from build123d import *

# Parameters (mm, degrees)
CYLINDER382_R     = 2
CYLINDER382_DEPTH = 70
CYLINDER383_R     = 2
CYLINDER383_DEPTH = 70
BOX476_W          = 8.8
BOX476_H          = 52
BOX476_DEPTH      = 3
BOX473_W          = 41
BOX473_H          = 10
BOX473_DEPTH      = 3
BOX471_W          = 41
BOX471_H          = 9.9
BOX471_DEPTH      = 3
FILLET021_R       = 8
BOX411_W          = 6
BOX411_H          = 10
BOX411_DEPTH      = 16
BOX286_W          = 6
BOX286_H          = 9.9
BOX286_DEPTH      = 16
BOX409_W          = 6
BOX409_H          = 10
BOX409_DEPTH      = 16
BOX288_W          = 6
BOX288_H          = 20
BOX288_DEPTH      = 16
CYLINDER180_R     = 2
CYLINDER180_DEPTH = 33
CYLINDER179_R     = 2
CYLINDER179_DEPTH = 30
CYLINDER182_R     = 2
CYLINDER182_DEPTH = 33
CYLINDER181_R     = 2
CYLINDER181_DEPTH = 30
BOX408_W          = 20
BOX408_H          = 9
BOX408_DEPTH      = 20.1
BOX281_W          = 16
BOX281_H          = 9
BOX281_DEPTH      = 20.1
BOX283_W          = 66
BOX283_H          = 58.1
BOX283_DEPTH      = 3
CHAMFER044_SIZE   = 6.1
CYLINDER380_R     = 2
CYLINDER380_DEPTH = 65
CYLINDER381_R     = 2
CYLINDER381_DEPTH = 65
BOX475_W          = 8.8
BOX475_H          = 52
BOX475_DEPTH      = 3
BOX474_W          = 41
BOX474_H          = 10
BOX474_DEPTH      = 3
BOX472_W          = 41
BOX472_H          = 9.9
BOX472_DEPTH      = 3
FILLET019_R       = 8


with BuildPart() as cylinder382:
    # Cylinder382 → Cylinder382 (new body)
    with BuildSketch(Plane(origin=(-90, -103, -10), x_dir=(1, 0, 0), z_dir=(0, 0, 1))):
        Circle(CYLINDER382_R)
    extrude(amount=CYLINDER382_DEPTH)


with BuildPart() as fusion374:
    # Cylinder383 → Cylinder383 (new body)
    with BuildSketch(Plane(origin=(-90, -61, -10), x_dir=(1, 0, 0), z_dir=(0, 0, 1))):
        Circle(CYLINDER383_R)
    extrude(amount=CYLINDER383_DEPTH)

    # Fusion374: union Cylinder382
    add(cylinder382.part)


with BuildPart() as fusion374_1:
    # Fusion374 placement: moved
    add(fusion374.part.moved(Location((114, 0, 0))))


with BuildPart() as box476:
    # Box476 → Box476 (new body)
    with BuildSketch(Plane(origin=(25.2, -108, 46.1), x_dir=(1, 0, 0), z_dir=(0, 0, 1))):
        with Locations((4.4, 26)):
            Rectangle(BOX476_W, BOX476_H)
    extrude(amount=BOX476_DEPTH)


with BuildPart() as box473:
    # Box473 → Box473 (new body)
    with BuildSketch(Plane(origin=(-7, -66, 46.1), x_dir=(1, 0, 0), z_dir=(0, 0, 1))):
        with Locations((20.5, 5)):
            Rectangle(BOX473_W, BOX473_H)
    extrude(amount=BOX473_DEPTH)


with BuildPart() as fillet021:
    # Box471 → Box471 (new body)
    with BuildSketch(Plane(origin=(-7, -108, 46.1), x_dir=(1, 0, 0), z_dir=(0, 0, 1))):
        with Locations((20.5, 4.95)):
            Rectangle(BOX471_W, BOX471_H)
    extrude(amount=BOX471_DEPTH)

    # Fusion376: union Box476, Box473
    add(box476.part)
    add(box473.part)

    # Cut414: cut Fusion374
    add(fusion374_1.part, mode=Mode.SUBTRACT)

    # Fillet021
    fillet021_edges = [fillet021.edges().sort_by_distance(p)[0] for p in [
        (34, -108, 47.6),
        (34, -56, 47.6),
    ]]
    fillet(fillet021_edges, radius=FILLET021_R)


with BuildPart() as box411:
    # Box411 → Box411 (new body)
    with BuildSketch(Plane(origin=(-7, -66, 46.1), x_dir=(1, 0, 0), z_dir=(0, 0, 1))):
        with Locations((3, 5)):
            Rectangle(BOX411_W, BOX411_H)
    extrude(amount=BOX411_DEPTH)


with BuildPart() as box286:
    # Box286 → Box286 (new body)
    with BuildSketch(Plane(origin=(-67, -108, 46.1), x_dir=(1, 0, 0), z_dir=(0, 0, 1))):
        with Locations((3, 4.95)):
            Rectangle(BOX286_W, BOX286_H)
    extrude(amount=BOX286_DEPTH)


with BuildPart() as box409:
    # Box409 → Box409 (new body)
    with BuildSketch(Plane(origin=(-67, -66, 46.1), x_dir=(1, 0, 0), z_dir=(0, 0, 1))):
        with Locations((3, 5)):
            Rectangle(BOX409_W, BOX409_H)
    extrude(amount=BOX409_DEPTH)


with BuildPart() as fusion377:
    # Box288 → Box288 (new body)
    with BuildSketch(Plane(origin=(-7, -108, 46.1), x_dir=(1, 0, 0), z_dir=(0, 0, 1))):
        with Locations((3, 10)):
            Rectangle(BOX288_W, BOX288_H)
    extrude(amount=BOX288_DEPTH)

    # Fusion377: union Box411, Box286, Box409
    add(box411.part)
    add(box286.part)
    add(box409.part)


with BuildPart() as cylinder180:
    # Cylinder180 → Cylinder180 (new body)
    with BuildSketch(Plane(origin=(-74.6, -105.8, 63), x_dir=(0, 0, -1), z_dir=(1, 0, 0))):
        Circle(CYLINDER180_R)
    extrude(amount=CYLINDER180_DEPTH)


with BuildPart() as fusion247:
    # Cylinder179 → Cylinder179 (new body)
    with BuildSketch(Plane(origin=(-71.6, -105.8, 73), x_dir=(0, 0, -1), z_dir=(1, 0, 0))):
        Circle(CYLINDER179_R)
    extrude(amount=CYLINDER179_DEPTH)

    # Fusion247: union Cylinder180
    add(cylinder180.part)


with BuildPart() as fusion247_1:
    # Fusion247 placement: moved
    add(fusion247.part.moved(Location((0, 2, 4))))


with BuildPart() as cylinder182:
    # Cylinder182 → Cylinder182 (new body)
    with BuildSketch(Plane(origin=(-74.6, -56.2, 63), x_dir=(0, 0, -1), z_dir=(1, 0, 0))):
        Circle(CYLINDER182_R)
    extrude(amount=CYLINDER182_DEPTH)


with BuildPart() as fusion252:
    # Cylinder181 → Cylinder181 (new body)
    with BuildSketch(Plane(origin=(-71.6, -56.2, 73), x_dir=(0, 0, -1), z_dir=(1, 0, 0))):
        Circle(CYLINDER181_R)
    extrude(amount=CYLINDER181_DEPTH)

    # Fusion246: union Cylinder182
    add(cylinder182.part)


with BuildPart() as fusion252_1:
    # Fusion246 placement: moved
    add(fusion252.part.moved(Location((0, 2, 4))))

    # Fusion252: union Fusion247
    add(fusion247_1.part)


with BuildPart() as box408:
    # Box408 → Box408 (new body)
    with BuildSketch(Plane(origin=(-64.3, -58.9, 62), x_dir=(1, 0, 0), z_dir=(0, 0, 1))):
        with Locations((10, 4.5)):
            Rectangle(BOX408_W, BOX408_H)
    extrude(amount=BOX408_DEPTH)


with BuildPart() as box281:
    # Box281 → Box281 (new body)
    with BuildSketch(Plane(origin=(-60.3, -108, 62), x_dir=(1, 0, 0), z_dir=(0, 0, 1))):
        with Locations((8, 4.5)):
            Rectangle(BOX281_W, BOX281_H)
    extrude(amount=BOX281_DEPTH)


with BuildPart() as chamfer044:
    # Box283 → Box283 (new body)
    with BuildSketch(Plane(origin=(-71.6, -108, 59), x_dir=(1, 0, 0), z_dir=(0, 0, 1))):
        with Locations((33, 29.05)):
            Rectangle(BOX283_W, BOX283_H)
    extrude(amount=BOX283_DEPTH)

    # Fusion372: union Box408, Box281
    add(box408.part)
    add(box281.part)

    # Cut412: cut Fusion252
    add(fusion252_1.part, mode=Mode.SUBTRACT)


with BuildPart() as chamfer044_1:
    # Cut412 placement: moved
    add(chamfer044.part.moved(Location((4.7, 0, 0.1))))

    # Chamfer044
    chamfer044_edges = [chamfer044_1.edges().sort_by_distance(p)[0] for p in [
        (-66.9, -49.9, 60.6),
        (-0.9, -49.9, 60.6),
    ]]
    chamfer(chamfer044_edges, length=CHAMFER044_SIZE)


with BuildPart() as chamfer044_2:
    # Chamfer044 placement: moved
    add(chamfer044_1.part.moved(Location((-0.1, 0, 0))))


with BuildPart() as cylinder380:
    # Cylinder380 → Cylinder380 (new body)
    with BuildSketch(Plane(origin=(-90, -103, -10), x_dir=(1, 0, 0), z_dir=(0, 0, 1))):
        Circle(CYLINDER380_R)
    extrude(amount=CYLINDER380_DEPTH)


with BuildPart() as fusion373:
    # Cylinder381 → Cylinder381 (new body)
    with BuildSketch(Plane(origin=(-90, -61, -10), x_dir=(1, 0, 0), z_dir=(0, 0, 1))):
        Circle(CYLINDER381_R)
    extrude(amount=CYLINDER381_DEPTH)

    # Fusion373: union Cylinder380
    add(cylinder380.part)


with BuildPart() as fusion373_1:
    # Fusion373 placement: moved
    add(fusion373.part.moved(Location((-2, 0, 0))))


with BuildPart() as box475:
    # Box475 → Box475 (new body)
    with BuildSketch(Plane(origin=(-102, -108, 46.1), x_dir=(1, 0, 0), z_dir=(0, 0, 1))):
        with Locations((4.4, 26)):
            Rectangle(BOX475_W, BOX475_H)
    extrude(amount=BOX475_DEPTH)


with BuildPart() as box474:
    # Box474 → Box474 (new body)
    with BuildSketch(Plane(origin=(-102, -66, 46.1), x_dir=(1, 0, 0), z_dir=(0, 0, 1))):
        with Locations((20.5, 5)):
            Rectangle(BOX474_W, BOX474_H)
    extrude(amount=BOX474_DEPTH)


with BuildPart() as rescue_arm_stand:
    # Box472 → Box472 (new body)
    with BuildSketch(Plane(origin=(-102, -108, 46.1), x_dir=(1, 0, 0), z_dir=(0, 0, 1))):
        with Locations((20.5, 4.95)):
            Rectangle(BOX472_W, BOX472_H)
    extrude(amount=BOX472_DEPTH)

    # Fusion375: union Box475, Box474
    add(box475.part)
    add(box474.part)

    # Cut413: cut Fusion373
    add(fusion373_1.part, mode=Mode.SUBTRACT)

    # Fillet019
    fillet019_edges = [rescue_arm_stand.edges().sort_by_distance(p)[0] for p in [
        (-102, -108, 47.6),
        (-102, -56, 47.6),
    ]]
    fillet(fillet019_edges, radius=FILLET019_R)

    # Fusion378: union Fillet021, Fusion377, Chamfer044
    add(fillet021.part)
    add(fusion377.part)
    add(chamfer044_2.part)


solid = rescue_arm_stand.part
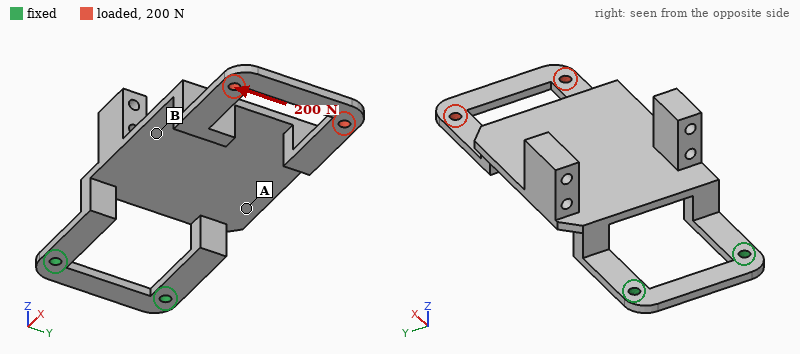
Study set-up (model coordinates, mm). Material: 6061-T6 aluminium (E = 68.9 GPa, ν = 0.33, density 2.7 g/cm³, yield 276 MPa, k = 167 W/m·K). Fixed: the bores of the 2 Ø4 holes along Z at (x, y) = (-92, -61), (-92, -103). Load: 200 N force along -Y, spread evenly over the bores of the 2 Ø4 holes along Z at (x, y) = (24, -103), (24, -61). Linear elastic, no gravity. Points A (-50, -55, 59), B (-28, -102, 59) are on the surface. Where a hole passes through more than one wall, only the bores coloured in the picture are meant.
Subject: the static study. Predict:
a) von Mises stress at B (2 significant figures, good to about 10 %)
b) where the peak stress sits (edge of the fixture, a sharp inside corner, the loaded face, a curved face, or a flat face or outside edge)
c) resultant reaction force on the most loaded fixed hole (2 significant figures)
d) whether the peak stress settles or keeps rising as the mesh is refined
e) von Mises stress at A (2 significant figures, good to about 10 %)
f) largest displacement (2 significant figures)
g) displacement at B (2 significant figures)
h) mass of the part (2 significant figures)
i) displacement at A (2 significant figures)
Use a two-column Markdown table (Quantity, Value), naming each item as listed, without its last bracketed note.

| Quantity | Value |
|---|---|
| von Mises stress at B | 42 MPa |
| where the peak stress sits | edge of the fixture |
| resultant reaction force on the most loaded fixed hole | 390 N |
| whether the peak stress settles or keeps rising as the mesh is refined | keeps rising |
| von Mises stress at A | 16 MPa |
| largest displacement | 1.3 mm |
| displacement at B | 0.46 mm |
| mass of the part | 71 g |
| displacement at A | 0.42 mm |
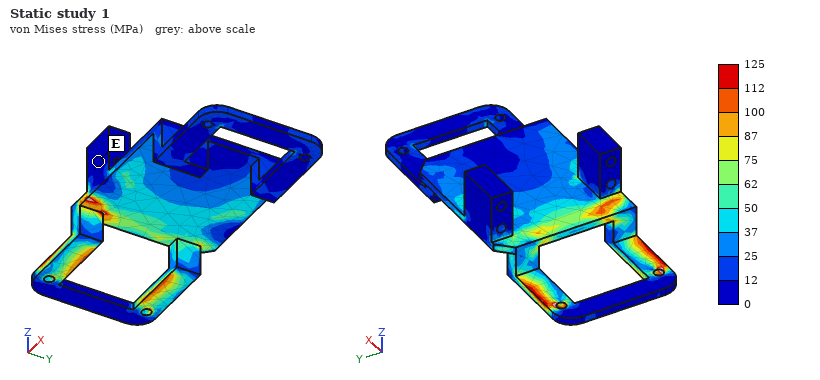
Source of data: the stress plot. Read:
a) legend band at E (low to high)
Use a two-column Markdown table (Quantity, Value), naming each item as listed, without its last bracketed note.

| Quantity | Value |
|---|---|
| legend band at E | 0 to 12 MPa |
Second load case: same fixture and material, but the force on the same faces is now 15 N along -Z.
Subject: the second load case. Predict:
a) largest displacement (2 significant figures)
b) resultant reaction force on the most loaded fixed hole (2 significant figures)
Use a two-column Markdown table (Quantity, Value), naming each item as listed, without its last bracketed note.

| Quantity | Value |
|---|---|
| largest displacement | 1.8 mm |
| resultant reaction force on the most loaded fixed hole | 11 N |
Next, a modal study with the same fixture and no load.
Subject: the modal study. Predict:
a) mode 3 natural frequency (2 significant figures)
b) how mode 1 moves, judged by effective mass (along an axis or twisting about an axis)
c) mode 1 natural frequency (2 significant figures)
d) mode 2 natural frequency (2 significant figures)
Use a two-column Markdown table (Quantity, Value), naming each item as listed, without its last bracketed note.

| Quantity | Value |
|---|---|
| mode 3 natural frequency | 690 Hz |
| how mode 1 moves, judged by effective mass | along Z |
| mode 1 natural frequency | 110 Hz |
| mode 2 natural frequency | 480 Hz |
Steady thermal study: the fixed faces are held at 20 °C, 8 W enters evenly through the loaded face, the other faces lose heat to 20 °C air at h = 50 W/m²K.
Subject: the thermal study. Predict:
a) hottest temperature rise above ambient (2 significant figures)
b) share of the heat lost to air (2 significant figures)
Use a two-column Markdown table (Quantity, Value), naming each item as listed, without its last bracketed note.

| Quantity | Value |
|---|---|
| hottest temperature rise above ambient | 29 K |
| share of the heat lost to air | 86 % |
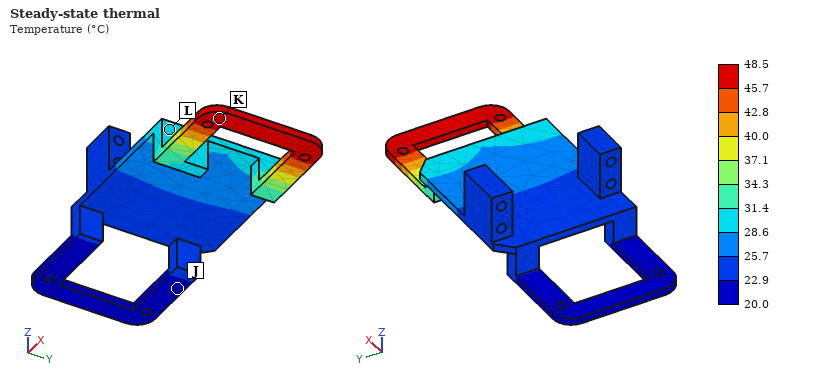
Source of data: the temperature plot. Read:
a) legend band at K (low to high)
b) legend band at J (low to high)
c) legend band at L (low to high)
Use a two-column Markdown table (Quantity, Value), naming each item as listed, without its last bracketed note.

| Quantity | Value |
|---|---|
| legend band at K | 45.7 to 48.5 °C |
| legend band at J | 20.0 to 22.9 °C |
| legend band at L | 28.6 to 31.4 °C |
